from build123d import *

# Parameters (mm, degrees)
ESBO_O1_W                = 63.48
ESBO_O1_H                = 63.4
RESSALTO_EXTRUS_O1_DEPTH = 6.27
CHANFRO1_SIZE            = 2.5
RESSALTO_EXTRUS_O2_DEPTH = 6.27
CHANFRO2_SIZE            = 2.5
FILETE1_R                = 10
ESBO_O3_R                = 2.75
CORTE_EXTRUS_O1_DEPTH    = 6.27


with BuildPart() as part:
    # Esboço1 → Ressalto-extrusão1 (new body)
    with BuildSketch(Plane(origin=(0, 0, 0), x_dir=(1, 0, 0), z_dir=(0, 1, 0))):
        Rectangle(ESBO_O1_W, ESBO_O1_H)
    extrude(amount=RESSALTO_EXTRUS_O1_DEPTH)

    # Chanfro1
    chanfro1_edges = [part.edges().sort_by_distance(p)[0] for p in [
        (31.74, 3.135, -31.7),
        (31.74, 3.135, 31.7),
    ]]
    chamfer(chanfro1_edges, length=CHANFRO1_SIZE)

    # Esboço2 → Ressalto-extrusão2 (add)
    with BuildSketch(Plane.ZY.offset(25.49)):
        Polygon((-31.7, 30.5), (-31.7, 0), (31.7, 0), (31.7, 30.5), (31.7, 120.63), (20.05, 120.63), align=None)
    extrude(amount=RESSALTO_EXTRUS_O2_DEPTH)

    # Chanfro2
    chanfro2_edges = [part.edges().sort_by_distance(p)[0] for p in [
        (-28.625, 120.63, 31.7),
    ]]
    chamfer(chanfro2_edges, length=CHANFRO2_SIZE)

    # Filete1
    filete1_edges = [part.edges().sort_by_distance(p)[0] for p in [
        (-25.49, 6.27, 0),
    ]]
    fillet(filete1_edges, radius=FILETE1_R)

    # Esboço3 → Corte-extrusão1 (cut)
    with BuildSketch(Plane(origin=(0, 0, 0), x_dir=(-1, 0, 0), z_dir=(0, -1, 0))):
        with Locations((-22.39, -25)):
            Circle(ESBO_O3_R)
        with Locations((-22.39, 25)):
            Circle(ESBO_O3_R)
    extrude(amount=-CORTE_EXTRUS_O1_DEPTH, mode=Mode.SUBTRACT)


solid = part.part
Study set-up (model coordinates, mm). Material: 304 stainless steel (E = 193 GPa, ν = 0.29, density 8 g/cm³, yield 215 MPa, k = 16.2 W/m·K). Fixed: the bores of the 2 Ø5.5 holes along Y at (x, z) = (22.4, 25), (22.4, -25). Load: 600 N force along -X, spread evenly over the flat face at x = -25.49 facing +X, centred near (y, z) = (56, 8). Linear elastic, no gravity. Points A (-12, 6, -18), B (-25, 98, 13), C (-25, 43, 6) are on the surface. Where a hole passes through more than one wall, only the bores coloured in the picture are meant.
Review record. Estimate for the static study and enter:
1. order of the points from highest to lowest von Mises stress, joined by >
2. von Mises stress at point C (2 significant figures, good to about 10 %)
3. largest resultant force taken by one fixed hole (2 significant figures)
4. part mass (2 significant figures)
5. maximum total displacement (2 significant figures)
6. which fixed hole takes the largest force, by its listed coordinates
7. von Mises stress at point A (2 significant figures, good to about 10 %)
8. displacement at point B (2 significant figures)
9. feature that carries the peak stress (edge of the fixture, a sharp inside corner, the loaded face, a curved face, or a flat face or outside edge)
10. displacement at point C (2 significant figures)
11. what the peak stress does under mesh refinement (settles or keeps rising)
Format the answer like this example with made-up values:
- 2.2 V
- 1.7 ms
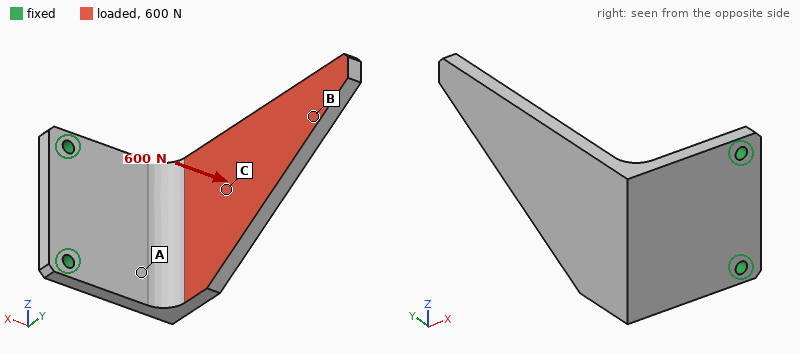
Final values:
- A > C > B
- 31 MPa
- 410 N
- 460 g
- 1.1 mm
- (22.4, 25)
- 71 MPa
- 0.82 mm
- edge of the fixture
- 0.32 mm
- keeps rising
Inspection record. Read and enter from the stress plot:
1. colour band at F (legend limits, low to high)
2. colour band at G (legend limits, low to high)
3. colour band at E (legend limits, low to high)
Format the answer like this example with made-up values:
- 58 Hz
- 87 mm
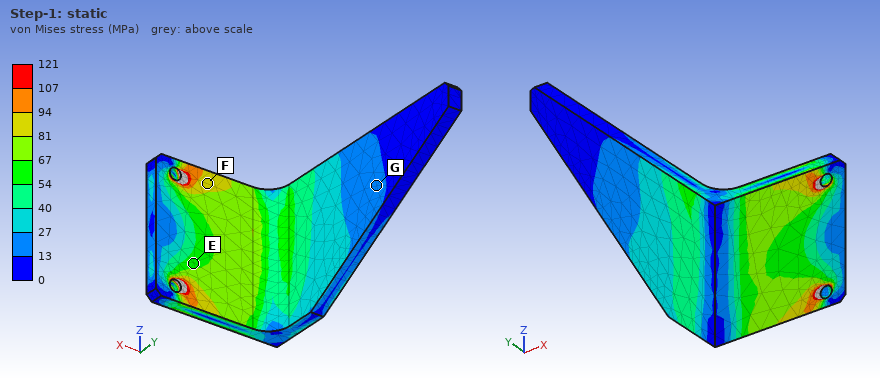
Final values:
- 81 to 94 MPa
- 13 to 27 MPa
- 54 to 67 MPa
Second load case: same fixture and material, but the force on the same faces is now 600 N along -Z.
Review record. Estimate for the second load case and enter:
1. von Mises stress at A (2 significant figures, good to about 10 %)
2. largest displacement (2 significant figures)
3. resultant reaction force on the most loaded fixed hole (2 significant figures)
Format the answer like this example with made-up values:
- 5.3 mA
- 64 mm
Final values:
- 46 MPa
- 0.26 mm
- 890 N
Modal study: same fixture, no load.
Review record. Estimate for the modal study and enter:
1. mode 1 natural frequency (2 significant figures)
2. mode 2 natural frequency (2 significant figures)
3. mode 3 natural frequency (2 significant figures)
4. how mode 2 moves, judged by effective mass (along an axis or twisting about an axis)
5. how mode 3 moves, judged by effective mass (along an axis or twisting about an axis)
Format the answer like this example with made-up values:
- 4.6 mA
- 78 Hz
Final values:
- 320 Hz
- 670 Hz
- 990 Hz
- along Z
- along Y
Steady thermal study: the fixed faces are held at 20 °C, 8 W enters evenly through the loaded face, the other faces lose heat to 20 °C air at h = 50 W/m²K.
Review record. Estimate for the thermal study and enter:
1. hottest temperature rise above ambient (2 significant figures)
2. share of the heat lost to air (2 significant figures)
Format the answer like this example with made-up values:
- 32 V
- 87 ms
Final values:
- 23 K
- 93 %
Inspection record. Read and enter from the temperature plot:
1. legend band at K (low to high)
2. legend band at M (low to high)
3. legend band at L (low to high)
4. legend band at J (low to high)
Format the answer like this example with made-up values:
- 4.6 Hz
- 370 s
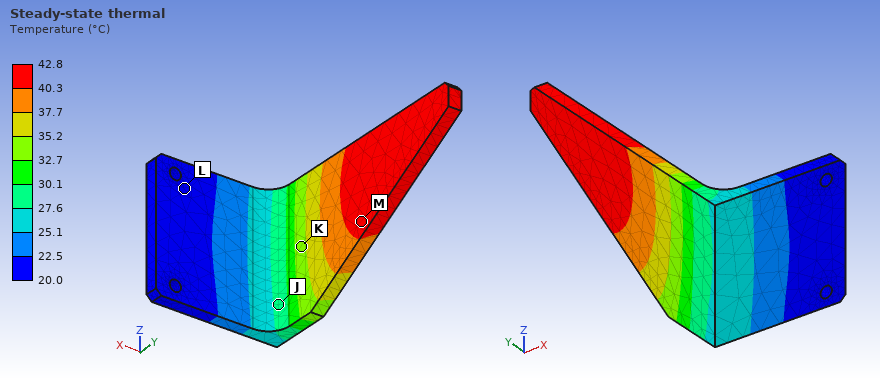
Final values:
- 32.7 to 35.2 °C
- 40.3 to 42.8 °C
- 20.0 to 22.5 °C
- 27.6 to 30.1 °C
